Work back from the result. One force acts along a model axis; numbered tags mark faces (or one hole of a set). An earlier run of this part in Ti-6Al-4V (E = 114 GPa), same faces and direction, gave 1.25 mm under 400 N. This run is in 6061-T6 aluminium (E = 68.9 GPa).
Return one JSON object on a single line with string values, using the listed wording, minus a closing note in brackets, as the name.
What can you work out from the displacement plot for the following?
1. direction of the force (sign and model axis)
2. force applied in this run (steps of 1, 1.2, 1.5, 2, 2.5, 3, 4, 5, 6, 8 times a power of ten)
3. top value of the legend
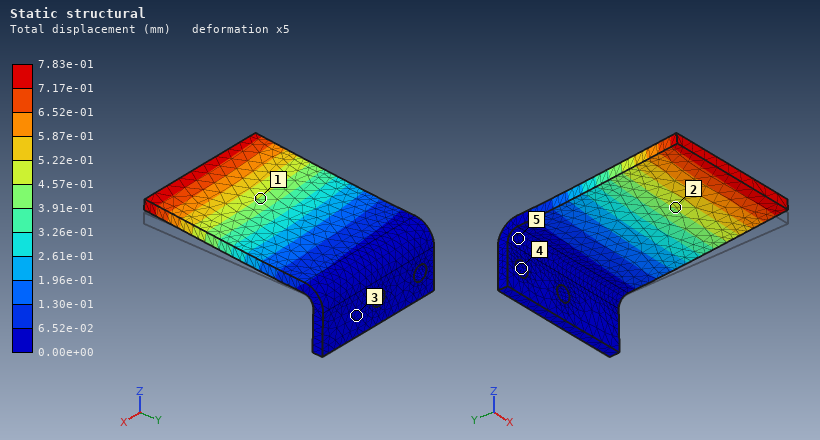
{"direction of the force": "+Z", "force applied in this run": "150 N", "top value of the legend": "7.83e-01 mm"}
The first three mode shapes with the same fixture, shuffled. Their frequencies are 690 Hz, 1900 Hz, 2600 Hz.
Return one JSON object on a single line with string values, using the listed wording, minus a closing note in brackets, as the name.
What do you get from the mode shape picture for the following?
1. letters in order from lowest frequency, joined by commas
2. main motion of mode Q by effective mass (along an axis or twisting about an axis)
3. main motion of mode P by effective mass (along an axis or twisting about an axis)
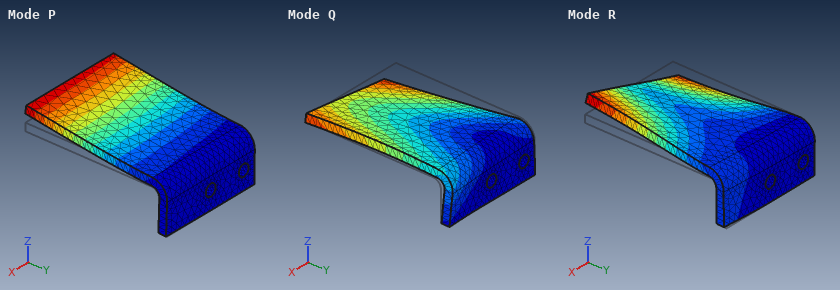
{"letters in order from lowest frequency, joined by commas": "P, Q, R", "main motion of mode Q by effective mass": "along X", "main motion of mode P by effective mass": "along Z"}
